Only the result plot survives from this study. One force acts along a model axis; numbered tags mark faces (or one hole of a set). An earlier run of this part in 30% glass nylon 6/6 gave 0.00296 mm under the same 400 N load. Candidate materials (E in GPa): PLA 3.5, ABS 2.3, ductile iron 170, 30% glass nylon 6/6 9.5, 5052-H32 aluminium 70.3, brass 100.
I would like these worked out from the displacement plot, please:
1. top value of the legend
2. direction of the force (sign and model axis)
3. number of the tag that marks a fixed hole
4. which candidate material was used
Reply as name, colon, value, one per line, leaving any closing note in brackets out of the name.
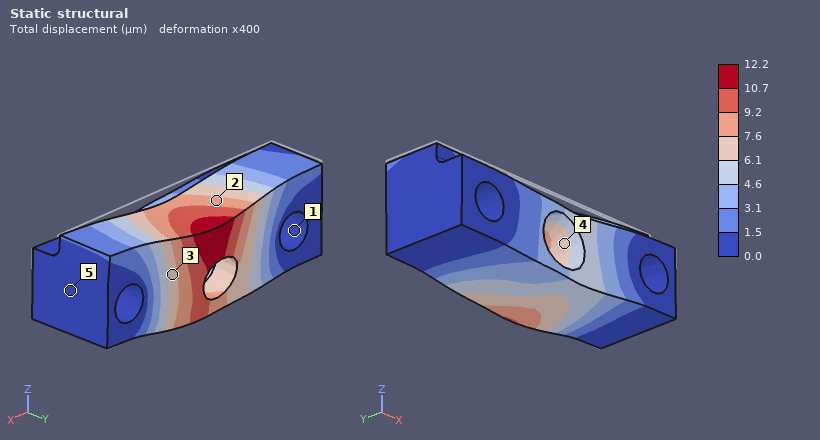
top value of the legend: 12.2 µm
direction of the force: -Z
number of the tag that marks a fixed hole: 1
which candidate material was used: ABS
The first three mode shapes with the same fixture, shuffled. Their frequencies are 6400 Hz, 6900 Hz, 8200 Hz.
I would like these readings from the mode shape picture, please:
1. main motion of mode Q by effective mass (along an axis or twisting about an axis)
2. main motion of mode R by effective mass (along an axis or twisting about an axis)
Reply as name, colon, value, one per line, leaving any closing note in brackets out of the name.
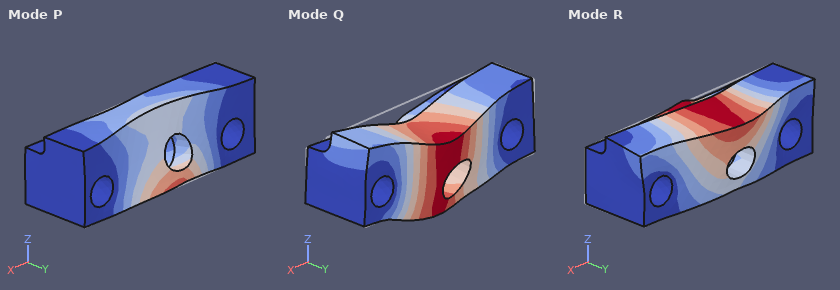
main motion of mode Q by effective mass: along Z
main motion of mode R by effective mass: along Y
